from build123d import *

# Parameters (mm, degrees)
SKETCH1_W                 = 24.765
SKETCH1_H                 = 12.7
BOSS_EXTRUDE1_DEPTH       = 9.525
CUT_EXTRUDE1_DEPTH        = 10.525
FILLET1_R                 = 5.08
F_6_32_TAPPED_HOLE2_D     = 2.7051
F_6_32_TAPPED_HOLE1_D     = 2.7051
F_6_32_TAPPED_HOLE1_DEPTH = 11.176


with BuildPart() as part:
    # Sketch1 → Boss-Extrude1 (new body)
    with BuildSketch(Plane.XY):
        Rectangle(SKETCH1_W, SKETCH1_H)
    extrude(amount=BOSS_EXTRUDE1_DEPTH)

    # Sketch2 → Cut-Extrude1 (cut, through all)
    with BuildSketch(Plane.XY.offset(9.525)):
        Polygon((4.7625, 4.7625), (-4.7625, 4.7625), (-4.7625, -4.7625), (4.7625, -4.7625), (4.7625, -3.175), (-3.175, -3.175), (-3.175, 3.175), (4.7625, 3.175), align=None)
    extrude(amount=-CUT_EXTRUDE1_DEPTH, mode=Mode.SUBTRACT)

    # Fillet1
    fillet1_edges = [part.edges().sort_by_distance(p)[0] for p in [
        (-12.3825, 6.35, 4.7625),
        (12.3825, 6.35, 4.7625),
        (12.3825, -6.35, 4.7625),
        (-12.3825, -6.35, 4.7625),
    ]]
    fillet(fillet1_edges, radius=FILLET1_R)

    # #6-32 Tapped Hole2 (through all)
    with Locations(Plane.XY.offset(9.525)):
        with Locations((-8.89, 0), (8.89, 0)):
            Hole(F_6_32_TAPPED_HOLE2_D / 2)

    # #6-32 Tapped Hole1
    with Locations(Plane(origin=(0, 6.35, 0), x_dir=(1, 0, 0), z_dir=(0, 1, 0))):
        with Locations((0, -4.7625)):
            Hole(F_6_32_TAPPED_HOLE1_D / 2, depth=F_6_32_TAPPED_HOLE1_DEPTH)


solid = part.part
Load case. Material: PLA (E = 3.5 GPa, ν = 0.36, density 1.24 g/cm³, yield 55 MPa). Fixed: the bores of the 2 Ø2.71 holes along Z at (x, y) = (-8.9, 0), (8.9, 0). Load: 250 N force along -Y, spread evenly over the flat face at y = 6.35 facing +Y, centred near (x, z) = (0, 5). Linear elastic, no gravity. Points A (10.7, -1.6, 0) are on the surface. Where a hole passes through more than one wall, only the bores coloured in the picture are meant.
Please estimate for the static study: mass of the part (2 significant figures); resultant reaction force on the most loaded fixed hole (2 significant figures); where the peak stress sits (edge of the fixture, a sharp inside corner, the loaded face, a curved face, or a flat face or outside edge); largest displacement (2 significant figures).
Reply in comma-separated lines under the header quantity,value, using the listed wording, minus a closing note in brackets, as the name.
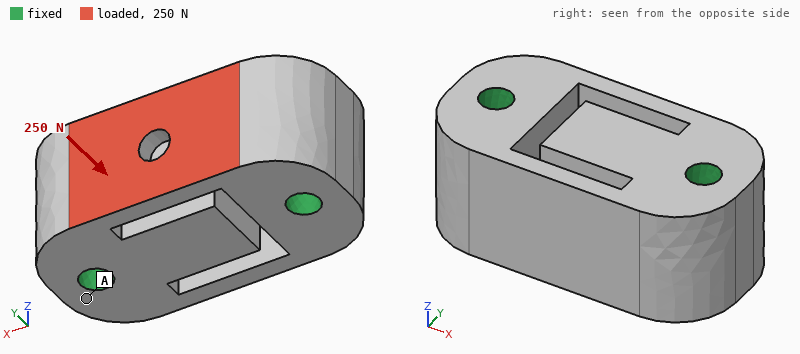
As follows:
quantity,value
mass of the part,2.8 g
resultant reaction force on the most loaded fixed hole,130 N
where the peak stress sits,the loaded face
largest displacement,89 µm
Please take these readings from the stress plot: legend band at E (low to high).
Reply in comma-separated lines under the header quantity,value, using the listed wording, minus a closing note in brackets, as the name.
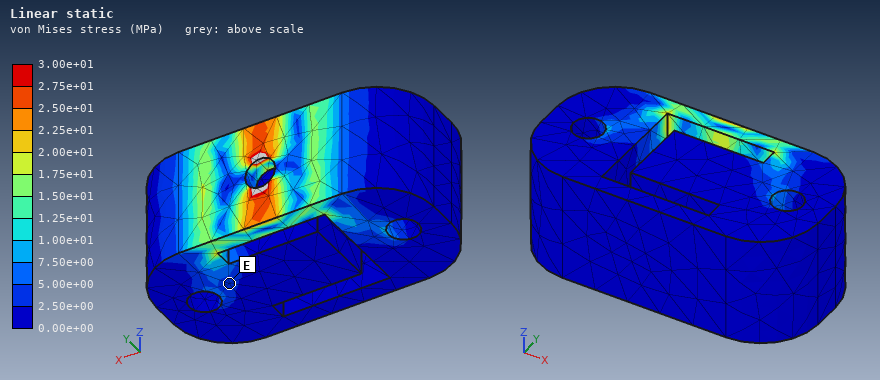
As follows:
quantity,value
legend band at E,2.50e+00 to 5.00e+00 MPa
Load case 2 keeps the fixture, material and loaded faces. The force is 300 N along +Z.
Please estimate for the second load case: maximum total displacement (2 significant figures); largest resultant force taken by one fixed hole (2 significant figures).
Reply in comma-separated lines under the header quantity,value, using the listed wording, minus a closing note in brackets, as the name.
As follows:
quantity,value
maximum total displacement,71 µm
largest resultant force taken by one fixed hole,150 N
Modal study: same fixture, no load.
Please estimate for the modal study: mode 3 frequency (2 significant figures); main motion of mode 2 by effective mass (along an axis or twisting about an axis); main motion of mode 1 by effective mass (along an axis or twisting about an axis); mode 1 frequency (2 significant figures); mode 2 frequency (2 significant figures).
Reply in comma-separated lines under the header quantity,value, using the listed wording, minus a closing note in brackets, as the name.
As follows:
quantity,value
mode 3 frequency,19 kHz
main motion of mode 2 by effective mass,along Z
main motion of mode 1 by effective mass,along Y
mode 1 frequency,11 kHz
mode 2 frequency,14 kHz
